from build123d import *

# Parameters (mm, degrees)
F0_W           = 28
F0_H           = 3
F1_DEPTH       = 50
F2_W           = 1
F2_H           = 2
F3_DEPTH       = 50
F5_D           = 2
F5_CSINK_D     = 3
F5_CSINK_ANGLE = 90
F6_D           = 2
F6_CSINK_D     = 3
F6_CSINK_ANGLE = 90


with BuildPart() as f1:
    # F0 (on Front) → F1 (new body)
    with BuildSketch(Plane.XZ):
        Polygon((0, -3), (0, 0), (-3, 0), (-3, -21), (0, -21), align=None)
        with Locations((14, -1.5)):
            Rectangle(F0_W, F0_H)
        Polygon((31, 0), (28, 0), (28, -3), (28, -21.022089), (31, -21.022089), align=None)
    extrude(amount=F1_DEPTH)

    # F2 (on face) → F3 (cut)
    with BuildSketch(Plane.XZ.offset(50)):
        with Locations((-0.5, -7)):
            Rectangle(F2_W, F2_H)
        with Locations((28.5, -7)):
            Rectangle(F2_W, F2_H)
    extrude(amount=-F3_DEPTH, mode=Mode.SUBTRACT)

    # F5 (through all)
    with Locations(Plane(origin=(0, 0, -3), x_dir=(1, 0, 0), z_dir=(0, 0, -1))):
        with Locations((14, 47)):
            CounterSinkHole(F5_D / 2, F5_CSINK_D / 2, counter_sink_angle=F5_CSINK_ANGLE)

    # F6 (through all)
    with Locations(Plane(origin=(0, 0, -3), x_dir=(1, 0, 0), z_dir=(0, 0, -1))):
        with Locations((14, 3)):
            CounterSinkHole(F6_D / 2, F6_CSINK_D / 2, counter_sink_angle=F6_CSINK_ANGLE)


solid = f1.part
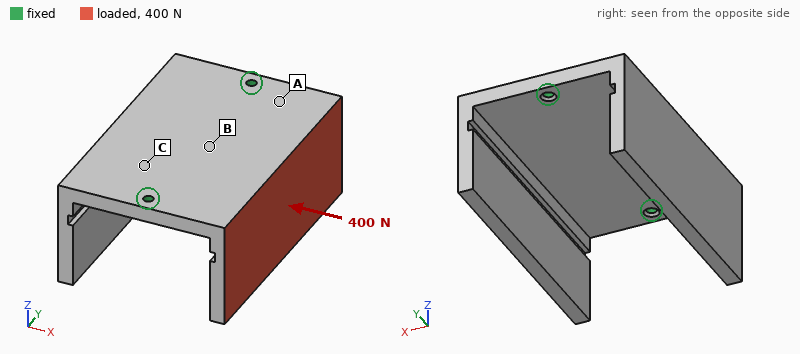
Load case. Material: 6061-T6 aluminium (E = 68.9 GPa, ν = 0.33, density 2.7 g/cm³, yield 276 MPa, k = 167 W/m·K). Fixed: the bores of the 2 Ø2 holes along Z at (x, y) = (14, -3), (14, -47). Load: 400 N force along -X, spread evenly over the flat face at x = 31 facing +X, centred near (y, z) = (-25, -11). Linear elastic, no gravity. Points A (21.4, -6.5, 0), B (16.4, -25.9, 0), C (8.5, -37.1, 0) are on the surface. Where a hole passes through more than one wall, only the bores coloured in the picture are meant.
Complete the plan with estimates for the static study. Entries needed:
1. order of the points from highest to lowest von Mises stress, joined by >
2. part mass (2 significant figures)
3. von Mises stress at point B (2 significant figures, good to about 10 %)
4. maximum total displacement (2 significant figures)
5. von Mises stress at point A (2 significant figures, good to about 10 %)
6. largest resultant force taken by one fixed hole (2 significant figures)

A > B > C
28 g
25 MPa
0.27 mm
47 MPa
200 N
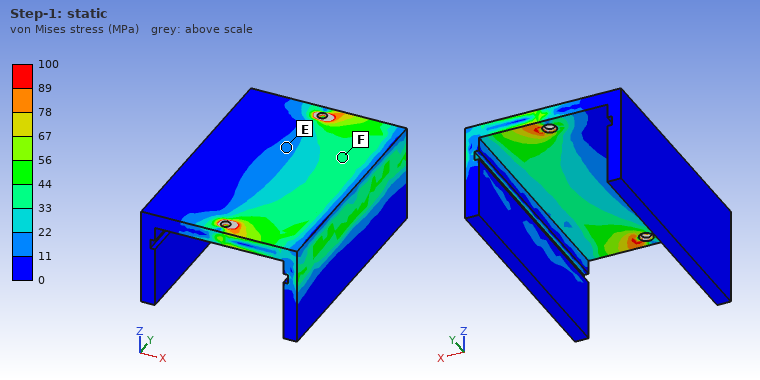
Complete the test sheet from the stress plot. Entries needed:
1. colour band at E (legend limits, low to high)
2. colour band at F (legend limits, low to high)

11 to 22 MPa
33 to 44 MPa
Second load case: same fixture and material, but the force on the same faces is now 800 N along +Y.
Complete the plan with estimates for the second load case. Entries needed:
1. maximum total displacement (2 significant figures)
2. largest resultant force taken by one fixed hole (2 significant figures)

98 µm
530 N
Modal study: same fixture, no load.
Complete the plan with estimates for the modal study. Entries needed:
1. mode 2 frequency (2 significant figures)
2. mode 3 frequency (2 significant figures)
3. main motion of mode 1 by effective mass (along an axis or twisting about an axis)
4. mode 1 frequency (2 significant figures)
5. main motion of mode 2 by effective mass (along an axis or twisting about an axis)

2600 Hz
3900 Hz
along X
1700 Hz
along Z
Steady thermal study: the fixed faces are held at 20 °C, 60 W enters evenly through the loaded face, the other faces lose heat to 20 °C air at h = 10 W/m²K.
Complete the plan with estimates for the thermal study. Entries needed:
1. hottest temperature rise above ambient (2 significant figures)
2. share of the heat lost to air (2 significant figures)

80 K
4.0 %
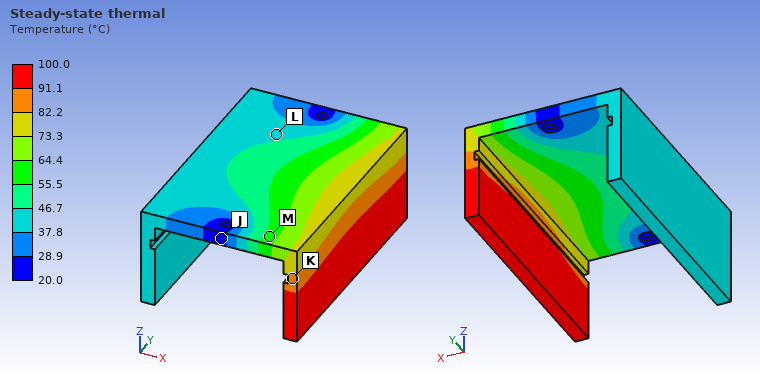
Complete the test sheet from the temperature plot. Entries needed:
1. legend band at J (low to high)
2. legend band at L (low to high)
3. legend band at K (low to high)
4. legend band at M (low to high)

20.0 to 28.9 °C
37.8 to 46.7 °C
82.2 to 91.1 °C
55.5 to 64.4 °C
